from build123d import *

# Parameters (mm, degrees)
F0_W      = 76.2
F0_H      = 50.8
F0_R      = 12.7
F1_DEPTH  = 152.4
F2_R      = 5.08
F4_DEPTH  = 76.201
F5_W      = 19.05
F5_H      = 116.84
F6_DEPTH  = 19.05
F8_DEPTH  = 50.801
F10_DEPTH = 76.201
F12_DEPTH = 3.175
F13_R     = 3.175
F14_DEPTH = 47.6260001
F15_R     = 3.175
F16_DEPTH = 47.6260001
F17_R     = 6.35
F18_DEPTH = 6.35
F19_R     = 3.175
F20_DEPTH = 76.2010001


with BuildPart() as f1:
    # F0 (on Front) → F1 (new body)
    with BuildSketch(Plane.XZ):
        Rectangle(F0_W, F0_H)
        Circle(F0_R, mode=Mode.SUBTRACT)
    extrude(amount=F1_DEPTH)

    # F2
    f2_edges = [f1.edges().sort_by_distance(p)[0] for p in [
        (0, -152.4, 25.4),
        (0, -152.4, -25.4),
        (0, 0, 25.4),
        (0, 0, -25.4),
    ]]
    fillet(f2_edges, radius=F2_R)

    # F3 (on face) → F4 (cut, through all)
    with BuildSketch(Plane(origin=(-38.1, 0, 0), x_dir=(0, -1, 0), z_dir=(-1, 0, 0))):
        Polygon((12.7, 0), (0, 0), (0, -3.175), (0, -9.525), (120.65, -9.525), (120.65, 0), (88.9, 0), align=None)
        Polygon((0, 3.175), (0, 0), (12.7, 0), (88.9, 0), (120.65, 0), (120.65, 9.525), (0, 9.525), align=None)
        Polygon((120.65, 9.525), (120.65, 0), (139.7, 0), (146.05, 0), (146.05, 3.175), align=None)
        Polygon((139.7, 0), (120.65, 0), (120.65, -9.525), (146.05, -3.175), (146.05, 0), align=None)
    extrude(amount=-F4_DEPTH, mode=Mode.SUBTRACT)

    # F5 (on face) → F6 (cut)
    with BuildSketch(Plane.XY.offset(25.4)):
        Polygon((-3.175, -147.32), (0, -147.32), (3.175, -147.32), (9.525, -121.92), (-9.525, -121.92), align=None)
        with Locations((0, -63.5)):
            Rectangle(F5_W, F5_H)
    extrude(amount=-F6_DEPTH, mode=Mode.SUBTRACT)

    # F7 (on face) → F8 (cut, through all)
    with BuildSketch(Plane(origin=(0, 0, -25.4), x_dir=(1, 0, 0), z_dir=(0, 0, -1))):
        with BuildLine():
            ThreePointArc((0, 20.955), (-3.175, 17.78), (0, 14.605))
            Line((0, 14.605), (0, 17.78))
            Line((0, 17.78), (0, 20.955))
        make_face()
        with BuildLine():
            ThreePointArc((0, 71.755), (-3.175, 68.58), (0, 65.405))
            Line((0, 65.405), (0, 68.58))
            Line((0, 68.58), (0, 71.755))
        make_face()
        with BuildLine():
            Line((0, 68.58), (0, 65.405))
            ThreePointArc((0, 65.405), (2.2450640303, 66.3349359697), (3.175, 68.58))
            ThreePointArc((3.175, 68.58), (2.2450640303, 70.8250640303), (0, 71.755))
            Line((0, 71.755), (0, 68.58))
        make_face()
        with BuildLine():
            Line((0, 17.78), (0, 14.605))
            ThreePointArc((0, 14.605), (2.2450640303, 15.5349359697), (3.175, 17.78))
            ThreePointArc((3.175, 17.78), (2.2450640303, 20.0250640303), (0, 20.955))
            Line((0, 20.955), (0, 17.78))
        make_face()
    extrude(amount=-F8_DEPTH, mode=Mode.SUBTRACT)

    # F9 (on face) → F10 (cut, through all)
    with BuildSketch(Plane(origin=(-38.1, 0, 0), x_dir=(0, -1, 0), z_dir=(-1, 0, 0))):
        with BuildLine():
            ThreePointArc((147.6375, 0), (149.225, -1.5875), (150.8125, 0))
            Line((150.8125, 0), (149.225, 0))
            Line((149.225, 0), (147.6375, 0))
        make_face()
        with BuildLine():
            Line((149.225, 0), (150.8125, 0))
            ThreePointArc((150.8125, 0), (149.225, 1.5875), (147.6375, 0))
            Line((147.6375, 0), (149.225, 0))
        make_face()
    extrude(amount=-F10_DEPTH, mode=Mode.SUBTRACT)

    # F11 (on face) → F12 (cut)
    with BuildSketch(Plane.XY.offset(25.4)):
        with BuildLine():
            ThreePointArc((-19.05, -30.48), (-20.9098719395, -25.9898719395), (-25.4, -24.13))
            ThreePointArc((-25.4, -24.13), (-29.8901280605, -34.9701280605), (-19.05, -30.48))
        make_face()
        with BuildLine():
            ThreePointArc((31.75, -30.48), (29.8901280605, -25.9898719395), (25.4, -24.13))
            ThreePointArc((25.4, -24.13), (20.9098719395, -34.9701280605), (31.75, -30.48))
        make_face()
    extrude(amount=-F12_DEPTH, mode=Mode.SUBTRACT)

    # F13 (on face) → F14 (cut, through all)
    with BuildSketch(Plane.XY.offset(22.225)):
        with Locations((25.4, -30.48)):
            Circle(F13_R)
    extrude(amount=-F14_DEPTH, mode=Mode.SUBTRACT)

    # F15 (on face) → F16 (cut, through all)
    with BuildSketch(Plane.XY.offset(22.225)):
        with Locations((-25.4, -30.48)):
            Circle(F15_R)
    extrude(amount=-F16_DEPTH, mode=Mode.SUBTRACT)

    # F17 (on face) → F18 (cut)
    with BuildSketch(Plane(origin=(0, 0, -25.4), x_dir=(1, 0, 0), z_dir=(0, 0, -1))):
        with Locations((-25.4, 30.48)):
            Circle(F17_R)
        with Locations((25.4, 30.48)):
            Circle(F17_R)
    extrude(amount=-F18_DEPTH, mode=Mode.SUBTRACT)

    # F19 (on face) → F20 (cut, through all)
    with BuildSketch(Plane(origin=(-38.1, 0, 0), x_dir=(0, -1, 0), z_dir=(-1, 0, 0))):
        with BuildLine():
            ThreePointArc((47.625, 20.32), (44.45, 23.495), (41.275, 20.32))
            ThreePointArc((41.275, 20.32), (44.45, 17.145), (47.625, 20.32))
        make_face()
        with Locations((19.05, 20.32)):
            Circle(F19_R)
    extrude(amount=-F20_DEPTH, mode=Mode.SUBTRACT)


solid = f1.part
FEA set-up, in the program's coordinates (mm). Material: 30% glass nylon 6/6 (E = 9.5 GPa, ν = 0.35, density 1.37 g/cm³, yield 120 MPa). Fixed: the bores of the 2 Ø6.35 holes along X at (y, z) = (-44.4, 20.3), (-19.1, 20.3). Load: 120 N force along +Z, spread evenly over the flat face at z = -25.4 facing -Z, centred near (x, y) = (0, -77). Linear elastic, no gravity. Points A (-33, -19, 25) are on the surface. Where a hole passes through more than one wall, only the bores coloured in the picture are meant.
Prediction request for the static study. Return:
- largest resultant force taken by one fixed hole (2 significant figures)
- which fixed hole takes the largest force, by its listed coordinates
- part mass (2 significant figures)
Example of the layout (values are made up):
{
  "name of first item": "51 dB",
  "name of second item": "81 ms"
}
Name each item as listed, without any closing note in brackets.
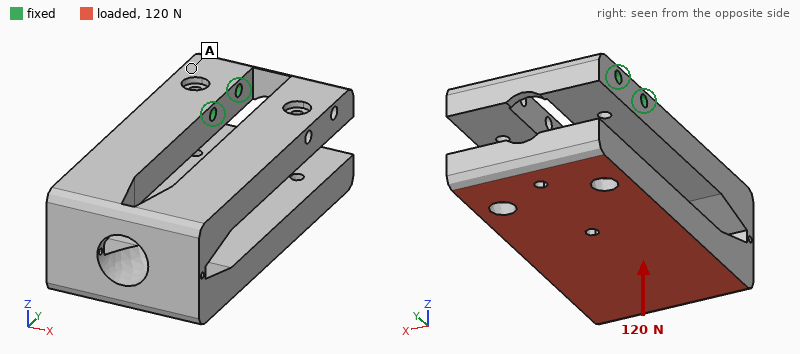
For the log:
{
  "largest resultant force taken by one fixed hole": "200 N",
  "which fixed hole takes the largest force, by its listed coordinates": "(-44.4, 20.3)",
  "part mass": "450 g"
}
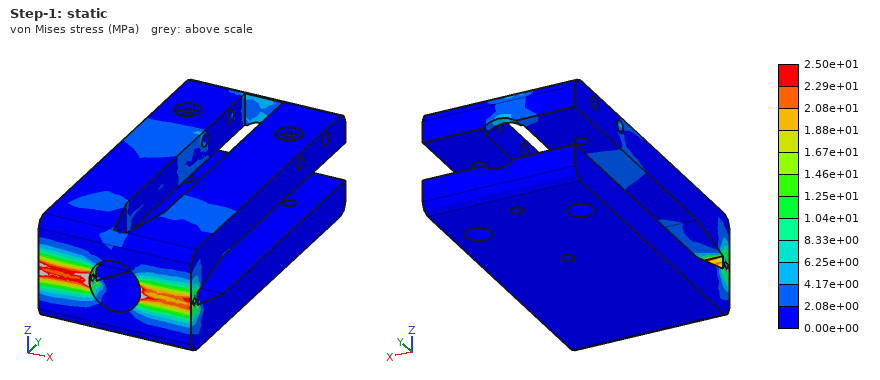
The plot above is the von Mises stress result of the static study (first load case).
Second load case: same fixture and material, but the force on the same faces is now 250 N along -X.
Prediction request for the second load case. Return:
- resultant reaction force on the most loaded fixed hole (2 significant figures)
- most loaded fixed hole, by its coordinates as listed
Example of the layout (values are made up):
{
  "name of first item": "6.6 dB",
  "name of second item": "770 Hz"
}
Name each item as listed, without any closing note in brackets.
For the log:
{
  "resultant reaction force on the most loaded fixed hole": "190 N",
  "most loaded fixed hole, by its coordinates as listed": "(-44.4, 20.3)"
}
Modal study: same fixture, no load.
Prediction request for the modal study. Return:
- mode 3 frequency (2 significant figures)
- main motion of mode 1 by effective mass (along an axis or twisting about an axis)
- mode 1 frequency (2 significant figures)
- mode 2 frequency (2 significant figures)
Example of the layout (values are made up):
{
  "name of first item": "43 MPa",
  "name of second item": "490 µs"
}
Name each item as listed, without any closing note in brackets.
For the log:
{
  "mode 3 frequency": "200 Hz",
  "main motion of mode 1 by effective mass": "along Z",
  "mode 1 frequency": "96 Hz",
  "mode 2 frequency": "160 Hz"
}
